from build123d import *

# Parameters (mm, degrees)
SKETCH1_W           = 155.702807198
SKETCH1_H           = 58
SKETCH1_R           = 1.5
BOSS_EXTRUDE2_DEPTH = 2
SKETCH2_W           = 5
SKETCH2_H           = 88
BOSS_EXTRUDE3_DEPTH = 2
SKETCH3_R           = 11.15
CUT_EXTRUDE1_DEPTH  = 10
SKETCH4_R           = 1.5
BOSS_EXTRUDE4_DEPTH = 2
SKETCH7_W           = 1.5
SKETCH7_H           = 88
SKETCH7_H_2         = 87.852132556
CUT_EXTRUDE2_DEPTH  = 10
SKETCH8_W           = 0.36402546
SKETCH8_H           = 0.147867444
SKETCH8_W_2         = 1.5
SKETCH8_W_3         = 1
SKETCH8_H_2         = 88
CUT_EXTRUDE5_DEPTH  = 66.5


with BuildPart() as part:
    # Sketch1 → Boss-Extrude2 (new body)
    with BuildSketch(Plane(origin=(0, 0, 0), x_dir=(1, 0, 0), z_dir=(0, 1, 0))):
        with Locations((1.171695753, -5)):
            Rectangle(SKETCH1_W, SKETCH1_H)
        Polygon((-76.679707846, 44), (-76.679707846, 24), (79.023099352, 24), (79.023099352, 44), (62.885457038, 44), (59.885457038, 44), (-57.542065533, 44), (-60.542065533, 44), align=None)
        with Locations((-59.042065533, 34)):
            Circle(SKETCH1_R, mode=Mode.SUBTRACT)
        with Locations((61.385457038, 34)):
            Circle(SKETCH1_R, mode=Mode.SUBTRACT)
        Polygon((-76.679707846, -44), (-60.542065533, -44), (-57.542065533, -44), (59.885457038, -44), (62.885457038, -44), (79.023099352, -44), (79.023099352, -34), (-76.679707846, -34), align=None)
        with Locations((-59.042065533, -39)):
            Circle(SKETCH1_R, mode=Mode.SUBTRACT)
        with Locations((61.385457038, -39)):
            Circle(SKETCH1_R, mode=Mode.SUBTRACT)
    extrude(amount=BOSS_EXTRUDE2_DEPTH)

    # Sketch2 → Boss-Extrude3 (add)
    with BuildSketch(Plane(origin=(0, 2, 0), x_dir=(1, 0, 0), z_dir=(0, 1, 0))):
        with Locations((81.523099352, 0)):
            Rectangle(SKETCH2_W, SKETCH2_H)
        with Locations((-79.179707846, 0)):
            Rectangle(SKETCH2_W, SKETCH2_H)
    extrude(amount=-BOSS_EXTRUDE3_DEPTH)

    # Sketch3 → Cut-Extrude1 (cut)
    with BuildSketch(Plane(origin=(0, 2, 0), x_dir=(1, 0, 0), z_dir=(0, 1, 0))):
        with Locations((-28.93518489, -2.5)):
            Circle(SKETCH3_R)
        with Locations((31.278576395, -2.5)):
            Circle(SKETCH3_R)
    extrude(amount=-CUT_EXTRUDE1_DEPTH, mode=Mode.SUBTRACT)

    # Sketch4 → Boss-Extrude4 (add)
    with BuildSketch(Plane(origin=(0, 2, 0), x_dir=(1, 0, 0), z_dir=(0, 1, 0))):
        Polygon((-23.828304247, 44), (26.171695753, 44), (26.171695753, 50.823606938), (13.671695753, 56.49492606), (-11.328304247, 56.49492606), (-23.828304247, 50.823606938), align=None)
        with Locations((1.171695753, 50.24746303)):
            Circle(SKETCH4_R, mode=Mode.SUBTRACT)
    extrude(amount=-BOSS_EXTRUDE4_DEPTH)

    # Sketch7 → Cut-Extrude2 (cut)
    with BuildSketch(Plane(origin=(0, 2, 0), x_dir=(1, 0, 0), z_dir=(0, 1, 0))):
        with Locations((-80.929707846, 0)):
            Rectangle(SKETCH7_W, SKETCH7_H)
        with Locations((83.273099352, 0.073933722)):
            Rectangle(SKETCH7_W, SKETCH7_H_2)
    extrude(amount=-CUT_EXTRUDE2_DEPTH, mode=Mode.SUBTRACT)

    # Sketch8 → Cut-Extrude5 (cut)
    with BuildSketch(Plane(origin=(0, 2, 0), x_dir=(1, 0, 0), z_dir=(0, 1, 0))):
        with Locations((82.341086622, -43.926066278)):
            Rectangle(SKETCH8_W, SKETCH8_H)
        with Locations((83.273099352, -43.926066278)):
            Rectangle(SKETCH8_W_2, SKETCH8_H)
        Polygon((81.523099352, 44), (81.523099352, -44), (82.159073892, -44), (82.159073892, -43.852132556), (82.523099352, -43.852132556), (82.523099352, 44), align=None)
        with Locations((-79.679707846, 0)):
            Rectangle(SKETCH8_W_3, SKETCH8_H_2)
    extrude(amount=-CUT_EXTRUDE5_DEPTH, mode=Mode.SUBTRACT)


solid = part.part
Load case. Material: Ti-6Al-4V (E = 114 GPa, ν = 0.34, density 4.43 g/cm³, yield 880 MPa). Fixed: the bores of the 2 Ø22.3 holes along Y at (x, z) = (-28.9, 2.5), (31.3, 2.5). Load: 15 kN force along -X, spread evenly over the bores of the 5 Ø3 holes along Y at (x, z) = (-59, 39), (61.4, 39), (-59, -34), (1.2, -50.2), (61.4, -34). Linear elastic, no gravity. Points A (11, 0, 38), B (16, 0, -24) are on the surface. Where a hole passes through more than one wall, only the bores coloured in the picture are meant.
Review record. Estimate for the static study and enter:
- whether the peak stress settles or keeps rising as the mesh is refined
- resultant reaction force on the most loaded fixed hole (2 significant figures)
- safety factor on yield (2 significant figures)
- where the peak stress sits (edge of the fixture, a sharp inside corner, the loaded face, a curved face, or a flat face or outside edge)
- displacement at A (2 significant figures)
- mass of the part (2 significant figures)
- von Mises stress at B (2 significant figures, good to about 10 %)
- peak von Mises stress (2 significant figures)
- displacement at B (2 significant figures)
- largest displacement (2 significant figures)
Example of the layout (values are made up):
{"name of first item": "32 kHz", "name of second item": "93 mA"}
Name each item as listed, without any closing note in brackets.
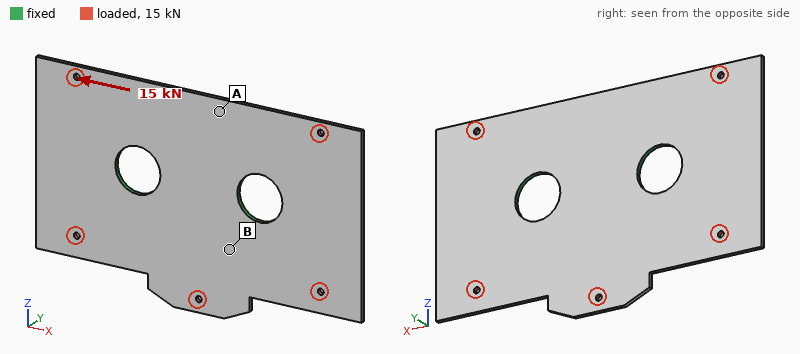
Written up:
{"whether the peak stress settles or keeps rising as the mesh is refined": "settles", "resultant reaction force on the most loaded fixed hole": "7.8 kN", "safety factor on yield": "3.0", "where the peak stress sits": "the loaded face", "displacement at A": "8.6 µm", "mass of the part": "120 g", "von Mises stress at B": "57 MPa", "peak von Mises stress": "290 MPa", "displacement at B": "16 µm", "largest displacement": "46 µm"}
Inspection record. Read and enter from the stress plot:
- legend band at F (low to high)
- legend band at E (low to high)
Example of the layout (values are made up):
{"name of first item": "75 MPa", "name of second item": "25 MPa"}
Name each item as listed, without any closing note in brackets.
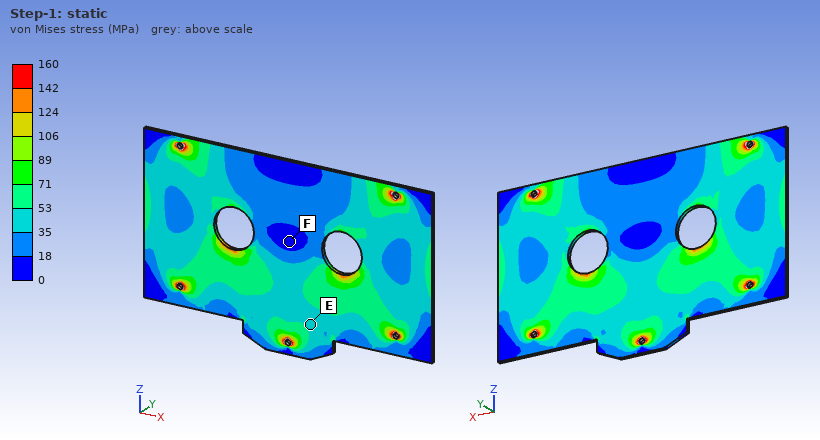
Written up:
{"legend band at F": "0 to 18 MPa", "legend band at E": "35 to 53 MPa"}
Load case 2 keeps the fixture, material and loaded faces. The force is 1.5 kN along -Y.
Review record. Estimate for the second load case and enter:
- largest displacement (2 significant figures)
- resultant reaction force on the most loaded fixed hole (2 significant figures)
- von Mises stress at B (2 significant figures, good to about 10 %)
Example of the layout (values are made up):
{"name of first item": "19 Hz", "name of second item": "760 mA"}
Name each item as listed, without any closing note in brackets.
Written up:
{"largest displacement": "1.9 mm", "resultant reaction force on the most loaded fixed hole": "750 N", "von Mises stress at B": "150 MPa"}
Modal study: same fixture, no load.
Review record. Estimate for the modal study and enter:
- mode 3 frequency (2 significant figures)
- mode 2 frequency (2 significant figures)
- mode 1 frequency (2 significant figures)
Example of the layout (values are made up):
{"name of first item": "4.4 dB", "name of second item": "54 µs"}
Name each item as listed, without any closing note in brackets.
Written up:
{"mode 3 frequency": "830 Hz", "mode 2 frequency": "780 Hz", "mode 1 frequency": "760 Hz"}
